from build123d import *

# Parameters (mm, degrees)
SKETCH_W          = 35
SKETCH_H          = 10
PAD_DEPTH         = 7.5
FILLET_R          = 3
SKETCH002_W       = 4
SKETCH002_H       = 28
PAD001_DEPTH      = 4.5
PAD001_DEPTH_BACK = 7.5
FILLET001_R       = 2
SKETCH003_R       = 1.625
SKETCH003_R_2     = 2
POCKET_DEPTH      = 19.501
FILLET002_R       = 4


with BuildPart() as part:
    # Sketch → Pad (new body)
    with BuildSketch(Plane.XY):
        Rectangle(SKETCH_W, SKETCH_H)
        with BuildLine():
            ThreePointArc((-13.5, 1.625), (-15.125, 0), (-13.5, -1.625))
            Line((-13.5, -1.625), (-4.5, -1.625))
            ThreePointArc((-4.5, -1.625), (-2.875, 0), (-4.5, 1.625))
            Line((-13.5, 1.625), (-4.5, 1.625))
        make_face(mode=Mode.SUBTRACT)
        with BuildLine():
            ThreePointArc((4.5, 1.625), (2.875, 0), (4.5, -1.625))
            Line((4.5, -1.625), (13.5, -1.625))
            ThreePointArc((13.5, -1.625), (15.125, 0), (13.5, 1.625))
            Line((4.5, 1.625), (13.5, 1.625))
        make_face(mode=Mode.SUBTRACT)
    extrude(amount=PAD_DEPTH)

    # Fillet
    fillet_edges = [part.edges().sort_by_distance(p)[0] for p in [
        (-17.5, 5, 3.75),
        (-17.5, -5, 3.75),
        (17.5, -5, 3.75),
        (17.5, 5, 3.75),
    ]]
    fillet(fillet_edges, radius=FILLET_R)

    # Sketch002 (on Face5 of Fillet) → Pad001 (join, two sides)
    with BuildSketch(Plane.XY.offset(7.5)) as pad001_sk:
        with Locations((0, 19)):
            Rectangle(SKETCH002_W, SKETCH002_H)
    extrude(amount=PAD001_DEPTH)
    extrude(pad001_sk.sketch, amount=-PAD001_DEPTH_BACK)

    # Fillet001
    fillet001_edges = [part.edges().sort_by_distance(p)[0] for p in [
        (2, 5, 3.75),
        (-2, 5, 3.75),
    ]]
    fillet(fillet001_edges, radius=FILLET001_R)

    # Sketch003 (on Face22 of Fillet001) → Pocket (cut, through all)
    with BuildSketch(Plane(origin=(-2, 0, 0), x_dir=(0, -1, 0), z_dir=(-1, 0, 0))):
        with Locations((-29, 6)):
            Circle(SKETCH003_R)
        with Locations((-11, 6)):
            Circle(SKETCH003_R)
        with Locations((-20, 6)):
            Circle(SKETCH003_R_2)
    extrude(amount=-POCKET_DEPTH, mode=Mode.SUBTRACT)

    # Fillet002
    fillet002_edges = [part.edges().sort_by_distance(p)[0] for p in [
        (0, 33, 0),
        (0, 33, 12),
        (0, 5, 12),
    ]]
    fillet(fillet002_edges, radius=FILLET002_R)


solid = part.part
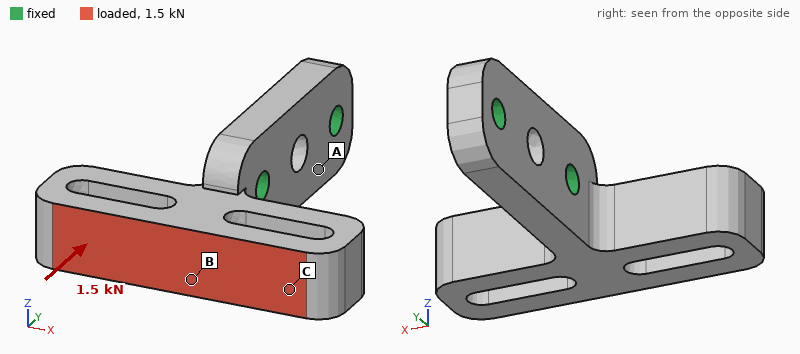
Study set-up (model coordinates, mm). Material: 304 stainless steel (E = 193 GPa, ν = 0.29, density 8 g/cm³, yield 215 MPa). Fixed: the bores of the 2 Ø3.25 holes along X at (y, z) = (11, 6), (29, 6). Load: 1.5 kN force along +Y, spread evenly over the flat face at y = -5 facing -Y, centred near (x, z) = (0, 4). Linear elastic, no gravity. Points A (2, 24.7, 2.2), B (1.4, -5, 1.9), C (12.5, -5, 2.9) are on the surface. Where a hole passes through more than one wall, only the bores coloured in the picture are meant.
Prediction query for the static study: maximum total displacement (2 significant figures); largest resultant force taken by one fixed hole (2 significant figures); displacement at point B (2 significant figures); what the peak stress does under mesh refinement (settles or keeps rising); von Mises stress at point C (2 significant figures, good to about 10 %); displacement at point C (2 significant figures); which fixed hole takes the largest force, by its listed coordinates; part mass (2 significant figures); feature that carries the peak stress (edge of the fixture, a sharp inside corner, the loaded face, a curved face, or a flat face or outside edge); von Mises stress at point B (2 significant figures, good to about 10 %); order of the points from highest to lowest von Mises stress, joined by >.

14 µm
1.4 kN
5.7 µm
keeps rising
34 MPa
12 µm
(11, 6)
26 g
edge of the fixture
78 MPa
B > C > A
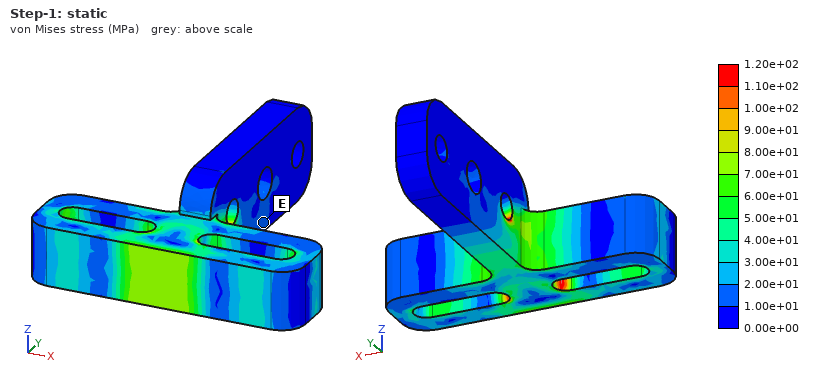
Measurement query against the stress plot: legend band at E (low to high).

1.00e+01 to 2.00e+01 MPa
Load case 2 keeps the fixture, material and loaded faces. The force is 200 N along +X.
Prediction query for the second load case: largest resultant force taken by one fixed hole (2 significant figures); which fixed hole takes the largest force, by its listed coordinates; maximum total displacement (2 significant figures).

220 N
(11, 6)
35 µm
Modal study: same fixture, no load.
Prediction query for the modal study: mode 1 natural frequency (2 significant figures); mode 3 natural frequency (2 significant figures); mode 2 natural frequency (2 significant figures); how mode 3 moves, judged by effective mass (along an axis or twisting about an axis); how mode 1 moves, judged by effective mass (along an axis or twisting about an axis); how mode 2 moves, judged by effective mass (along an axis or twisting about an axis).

3700 Hz
8900 Hz
5600 Hz
along Z
along X
twisting about Y
